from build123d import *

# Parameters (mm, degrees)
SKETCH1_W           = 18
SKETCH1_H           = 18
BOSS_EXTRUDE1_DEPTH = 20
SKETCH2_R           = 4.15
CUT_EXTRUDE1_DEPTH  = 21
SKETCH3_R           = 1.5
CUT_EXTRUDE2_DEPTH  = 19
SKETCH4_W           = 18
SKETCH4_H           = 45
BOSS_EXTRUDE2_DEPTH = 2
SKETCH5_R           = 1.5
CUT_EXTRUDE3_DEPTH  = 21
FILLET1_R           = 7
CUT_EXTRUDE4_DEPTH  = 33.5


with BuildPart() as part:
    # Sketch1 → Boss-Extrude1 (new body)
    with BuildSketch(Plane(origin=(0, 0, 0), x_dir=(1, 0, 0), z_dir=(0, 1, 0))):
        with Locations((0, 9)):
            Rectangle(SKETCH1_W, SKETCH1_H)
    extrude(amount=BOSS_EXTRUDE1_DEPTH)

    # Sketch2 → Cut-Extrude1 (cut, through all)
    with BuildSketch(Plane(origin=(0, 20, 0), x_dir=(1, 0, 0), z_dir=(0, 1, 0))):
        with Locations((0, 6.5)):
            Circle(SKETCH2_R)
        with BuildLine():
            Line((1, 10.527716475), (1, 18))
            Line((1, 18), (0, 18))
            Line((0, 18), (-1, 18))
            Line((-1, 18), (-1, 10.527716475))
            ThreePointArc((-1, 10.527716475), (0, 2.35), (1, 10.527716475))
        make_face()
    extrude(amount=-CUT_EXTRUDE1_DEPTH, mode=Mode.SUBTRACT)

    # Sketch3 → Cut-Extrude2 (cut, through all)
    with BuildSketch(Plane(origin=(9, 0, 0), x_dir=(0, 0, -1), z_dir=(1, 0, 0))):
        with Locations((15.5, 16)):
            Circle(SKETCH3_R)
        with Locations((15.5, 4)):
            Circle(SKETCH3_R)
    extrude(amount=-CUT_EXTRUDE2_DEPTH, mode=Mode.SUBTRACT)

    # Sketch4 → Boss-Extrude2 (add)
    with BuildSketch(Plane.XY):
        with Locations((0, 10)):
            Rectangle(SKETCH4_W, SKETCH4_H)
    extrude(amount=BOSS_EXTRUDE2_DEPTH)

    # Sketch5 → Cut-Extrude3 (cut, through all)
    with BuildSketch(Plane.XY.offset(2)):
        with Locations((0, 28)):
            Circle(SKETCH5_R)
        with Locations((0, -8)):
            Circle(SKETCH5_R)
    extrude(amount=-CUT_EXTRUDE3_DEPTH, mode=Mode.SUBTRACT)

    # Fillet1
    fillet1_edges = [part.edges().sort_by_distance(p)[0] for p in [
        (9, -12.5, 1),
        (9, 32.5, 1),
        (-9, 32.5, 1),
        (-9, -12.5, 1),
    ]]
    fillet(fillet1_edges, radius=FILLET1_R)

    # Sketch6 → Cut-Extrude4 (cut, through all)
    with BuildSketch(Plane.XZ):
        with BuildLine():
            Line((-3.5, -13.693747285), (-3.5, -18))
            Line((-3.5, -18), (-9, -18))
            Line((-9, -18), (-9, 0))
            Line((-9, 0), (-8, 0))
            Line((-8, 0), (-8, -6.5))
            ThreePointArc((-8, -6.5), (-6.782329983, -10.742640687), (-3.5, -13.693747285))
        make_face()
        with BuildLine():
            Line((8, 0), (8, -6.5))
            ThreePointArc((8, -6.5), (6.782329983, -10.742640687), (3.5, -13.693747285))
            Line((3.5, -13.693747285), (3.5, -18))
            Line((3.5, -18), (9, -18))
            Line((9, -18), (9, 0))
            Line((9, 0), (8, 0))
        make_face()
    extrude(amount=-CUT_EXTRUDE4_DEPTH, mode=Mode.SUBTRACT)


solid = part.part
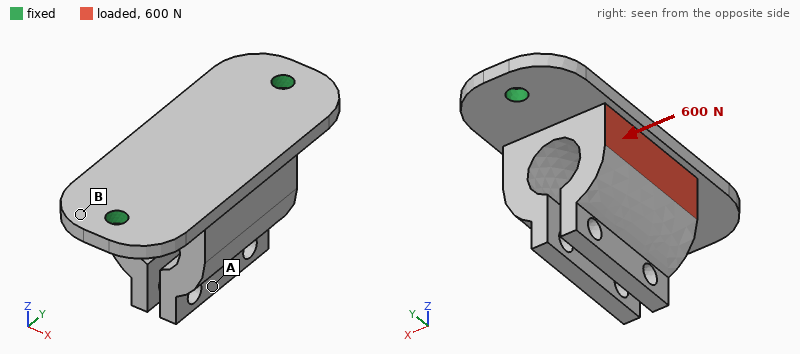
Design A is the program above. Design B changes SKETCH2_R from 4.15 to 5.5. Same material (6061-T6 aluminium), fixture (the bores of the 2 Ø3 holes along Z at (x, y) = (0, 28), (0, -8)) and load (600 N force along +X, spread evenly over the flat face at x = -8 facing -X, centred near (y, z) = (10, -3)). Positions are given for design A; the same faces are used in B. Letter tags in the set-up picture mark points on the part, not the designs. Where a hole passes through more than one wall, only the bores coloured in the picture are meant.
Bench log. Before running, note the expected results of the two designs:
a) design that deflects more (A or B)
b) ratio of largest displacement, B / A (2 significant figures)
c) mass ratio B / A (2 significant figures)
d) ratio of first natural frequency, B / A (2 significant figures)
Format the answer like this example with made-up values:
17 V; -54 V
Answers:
B; 1.2; 0.84; 1.0
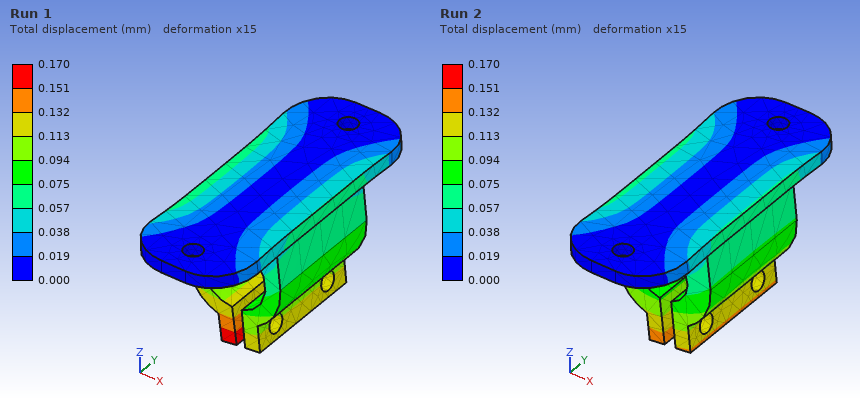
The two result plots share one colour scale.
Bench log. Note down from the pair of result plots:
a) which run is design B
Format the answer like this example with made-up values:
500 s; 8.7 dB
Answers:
Run 1
